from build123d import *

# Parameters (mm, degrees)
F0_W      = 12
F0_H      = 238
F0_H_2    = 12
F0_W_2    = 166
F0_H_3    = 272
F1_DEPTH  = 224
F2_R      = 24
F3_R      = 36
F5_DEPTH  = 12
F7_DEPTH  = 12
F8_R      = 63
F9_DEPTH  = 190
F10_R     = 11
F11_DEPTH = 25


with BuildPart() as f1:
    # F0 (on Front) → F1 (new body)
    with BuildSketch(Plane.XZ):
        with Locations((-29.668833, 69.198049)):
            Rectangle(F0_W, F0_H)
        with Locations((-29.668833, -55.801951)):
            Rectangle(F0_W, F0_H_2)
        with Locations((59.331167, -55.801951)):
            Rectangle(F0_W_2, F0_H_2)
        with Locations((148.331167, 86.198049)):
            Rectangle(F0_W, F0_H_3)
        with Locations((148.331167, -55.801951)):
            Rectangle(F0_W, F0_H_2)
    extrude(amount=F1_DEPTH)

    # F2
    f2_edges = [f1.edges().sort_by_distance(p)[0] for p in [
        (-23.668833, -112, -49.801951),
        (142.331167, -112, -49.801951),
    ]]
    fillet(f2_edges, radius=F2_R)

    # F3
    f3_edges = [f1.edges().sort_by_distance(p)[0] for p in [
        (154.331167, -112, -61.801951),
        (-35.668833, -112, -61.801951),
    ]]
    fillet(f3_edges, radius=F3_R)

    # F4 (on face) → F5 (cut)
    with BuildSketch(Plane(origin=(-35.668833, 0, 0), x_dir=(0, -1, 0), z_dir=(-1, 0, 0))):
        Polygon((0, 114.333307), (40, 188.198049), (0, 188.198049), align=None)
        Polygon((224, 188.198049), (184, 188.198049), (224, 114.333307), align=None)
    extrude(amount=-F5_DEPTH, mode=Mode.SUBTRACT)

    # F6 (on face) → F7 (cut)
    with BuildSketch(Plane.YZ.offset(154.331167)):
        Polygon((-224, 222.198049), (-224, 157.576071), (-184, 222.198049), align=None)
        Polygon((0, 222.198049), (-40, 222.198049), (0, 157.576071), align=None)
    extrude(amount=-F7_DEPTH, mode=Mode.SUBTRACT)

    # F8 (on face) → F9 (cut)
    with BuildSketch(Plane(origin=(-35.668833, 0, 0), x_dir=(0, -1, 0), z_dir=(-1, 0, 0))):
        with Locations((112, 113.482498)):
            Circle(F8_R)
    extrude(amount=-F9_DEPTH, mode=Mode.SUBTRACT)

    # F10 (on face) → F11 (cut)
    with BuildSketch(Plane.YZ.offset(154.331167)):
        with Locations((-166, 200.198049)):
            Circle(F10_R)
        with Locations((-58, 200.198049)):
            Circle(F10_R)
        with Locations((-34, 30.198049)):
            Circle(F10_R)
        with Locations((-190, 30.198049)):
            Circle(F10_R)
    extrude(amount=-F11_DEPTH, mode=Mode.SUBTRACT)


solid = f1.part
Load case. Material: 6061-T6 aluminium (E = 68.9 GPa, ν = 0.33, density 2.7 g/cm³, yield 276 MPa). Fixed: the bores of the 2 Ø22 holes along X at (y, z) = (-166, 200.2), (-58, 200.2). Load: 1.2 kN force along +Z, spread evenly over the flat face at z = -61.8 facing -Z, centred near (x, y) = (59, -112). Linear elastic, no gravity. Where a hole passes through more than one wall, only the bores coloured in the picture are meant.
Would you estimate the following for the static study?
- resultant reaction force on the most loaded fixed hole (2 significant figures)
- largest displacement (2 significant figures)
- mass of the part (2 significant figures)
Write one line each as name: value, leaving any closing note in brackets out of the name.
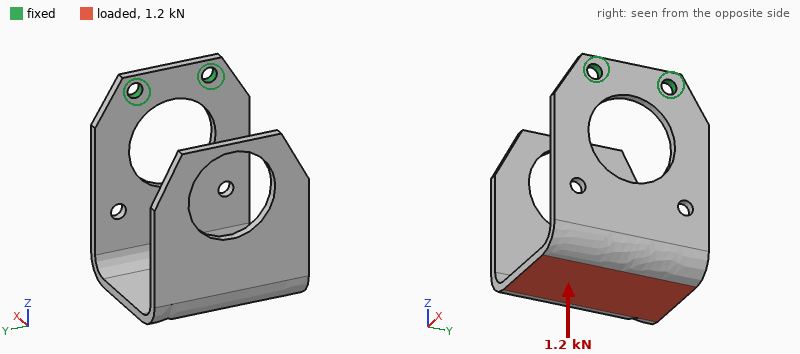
resultant reaction force on the most loaded fixed hole: 600 N
largest displacement: 4.6 mm
mass of the part: 3.9 kg
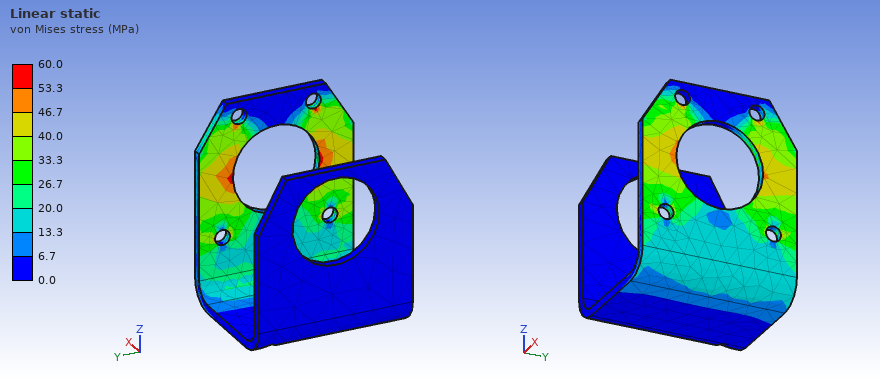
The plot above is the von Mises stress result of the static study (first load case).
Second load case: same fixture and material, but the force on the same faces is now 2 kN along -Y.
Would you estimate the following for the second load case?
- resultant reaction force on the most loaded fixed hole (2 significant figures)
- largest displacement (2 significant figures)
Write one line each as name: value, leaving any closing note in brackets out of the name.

resultant reaction force on the most loaded fixed hole: 3.6 kN
largest displacement: 3.3 mm
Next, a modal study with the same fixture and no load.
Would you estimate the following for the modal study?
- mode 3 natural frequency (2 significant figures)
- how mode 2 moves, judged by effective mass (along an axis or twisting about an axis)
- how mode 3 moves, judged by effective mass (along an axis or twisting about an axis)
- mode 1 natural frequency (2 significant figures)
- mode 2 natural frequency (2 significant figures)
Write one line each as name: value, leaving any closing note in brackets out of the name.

mode 3 natural frequency: 87 Hz
how mode 2 moves, judged by effective mass: along Y
how mode 3 moves, judged by effective mass: along X
mode 1 natural frequency: 38 Hz
mode 2 natural frequency: 64 Hz
